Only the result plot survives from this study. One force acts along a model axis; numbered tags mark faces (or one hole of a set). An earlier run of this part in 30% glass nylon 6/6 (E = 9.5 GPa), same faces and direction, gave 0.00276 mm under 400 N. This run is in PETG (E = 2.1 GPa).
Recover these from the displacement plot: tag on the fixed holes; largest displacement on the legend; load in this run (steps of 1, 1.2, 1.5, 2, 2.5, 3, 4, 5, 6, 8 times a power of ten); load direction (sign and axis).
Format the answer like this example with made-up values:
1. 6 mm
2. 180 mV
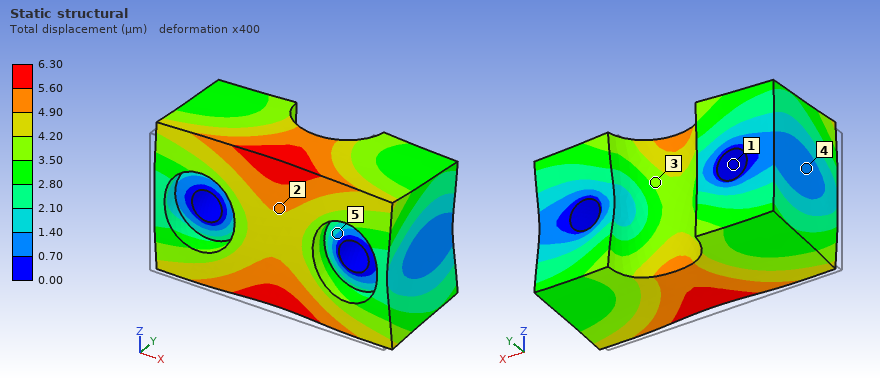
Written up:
1. 1
2. 6.30 µm
3. 200 N
4. +Y
